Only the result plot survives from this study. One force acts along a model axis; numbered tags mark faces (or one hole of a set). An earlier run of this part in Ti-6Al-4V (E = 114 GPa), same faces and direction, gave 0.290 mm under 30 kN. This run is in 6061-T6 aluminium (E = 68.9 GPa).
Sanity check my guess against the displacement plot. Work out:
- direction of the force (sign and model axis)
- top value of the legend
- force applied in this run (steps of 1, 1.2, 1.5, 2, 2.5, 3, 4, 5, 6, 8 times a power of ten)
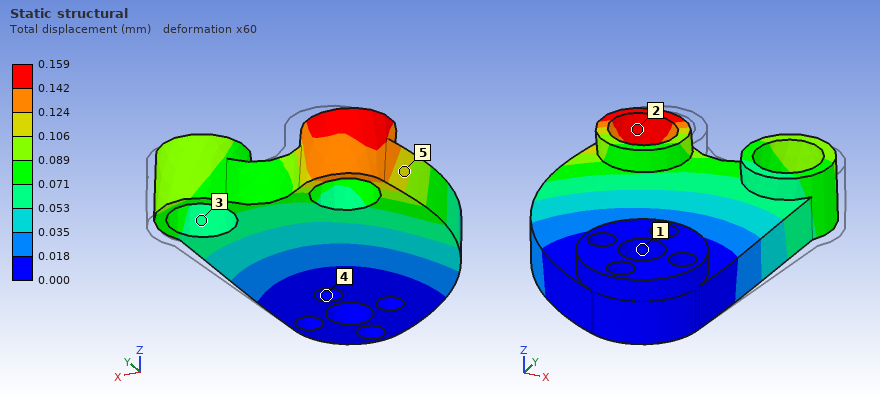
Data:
-X
0.159 mm
10 kN
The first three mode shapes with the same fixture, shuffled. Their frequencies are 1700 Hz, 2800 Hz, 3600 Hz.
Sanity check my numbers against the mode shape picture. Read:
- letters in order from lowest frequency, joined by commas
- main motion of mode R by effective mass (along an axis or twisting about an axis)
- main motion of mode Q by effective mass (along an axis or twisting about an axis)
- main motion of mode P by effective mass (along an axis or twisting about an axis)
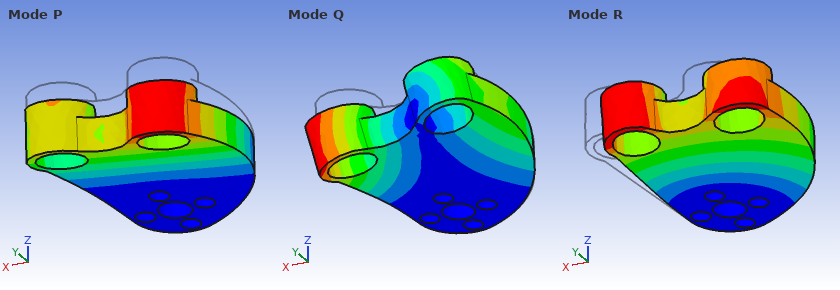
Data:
P, Q, R
along X
twisting about Y
along Z
